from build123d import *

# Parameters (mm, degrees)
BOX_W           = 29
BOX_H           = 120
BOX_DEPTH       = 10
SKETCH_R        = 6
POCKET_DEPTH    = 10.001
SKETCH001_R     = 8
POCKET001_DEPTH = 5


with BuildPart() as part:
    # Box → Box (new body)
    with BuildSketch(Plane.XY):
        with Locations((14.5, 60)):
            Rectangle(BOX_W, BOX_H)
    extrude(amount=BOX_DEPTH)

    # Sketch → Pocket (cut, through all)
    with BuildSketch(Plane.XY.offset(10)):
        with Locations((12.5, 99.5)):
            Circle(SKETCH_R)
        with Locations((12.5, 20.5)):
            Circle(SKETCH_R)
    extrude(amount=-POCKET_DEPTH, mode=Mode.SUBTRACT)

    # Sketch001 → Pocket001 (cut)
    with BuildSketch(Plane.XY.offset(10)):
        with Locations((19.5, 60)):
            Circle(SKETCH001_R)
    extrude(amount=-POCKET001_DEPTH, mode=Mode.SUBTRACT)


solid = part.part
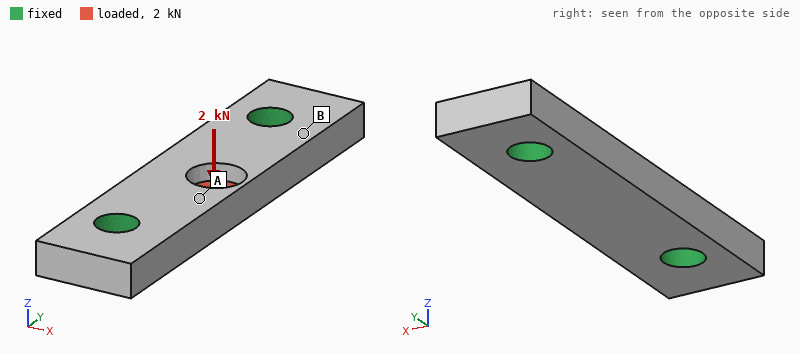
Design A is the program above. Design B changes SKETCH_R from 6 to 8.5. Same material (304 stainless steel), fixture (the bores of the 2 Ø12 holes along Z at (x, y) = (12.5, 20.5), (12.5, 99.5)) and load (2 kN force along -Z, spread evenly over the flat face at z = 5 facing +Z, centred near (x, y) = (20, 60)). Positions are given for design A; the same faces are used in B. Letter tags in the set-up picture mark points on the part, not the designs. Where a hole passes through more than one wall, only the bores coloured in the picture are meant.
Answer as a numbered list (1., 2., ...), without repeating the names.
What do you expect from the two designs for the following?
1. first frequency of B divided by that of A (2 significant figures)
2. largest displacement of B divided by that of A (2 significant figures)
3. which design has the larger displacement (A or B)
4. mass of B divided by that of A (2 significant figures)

1. 1.2
2. 0.81
3. A
4. 0.93
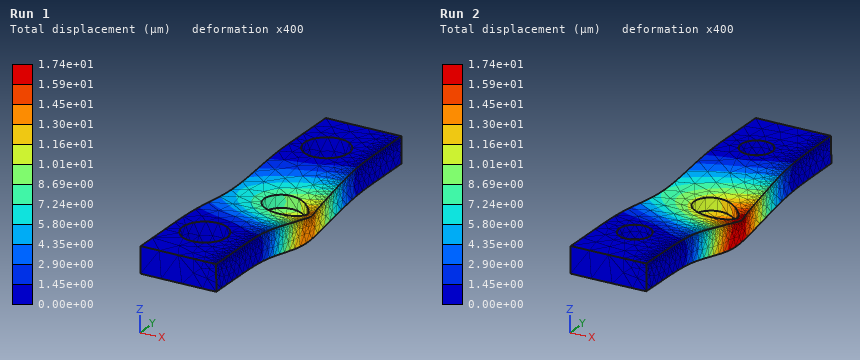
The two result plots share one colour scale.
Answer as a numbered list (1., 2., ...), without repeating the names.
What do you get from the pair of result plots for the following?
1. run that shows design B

1. Run 1
